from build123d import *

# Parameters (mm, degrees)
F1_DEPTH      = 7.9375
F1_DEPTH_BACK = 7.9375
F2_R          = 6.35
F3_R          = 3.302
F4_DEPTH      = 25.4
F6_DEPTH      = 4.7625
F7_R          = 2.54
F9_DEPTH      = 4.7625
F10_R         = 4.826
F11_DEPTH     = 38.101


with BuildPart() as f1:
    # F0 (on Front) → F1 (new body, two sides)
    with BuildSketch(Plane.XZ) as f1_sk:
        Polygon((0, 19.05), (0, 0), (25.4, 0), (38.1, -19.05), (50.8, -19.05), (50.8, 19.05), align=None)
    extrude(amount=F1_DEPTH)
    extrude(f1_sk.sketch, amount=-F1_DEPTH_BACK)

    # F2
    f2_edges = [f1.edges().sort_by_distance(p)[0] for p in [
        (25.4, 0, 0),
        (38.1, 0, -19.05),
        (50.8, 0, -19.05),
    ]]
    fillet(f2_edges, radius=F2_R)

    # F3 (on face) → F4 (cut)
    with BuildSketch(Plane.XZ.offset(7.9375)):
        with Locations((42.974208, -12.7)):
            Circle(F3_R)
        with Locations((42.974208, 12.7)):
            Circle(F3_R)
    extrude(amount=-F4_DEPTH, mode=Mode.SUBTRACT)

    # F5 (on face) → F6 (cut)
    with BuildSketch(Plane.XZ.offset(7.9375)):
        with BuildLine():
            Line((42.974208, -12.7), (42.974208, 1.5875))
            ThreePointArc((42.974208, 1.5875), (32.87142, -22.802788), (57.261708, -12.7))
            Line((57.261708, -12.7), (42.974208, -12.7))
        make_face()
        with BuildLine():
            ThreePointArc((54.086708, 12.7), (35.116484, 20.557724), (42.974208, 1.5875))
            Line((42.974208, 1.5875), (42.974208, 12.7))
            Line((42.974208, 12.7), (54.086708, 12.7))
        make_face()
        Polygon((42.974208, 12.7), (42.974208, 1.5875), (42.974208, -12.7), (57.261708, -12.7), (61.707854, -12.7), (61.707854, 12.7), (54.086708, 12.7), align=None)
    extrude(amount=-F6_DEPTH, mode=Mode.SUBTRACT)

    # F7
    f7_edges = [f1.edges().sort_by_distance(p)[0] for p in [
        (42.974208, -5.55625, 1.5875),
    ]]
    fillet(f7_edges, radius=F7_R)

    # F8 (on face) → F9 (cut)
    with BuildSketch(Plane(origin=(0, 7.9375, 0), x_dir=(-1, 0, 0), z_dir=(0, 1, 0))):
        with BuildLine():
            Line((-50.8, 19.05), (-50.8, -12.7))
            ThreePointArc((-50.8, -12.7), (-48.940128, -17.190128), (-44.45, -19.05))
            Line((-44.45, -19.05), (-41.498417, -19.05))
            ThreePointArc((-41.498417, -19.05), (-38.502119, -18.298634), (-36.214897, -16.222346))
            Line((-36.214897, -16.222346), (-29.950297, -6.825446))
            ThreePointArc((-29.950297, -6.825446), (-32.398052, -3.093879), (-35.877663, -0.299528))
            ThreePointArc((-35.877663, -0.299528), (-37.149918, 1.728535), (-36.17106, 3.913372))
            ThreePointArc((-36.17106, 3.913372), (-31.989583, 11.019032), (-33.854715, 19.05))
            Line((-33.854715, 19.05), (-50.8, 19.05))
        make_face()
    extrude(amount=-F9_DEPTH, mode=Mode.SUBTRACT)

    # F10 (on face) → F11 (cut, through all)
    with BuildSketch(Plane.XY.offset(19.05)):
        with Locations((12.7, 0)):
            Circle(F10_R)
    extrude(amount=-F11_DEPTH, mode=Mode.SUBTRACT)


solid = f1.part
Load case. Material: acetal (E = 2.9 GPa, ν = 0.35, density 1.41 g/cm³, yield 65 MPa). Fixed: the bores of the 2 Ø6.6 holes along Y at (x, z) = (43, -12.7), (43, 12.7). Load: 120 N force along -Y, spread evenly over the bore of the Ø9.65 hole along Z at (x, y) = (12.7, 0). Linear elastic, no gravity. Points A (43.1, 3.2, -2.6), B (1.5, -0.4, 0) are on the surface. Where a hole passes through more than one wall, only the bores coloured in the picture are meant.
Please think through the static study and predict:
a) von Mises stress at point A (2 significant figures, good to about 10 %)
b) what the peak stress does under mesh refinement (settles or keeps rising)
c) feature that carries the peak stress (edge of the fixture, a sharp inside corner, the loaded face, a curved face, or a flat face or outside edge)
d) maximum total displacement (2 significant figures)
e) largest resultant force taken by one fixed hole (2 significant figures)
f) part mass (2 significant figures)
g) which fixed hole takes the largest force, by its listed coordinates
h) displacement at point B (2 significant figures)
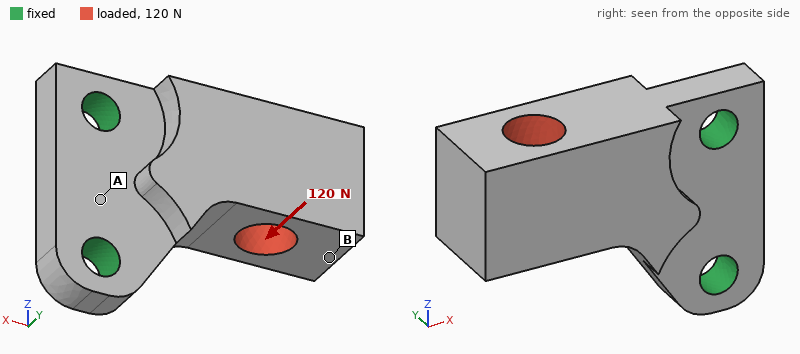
4.7 MPa
keeps rising
edge of the fixture
0.64 mm
98 N
18 g
(43, 12.7)
0.60 mm
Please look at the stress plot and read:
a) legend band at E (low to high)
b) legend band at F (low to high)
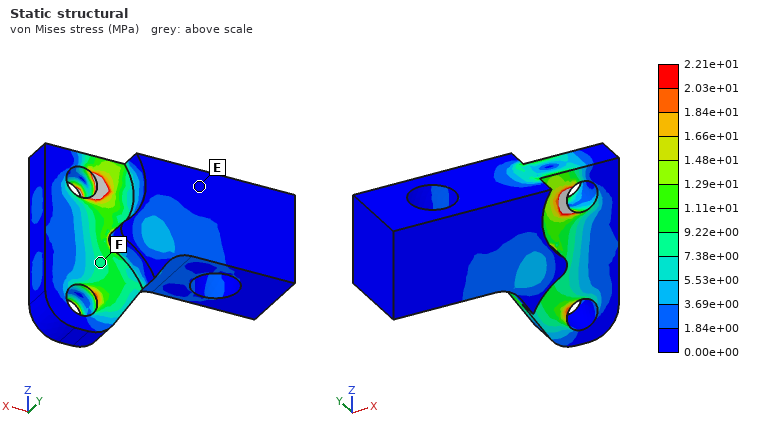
0.00e+00 to 1.84e+00 MPa
7.38e+00 to 9.22e+00 MPa
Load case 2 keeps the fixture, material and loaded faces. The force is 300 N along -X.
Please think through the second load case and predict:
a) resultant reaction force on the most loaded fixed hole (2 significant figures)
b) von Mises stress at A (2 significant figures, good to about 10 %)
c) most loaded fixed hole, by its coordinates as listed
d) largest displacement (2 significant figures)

260 N
0.60 MPa
(43, 12.7)
28 µm
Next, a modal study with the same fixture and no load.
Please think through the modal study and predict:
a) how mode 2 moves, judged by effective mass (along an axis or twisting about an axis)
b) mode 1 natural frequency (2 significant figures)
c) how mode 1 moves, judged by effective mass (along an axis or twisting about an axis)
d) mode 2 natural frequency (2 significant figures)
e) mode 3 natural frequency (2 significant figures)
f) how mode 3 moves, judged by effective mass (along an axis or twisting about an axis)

along Z
830 Hz
along Y
2400 Hz
3900 Hz
twisting about X
